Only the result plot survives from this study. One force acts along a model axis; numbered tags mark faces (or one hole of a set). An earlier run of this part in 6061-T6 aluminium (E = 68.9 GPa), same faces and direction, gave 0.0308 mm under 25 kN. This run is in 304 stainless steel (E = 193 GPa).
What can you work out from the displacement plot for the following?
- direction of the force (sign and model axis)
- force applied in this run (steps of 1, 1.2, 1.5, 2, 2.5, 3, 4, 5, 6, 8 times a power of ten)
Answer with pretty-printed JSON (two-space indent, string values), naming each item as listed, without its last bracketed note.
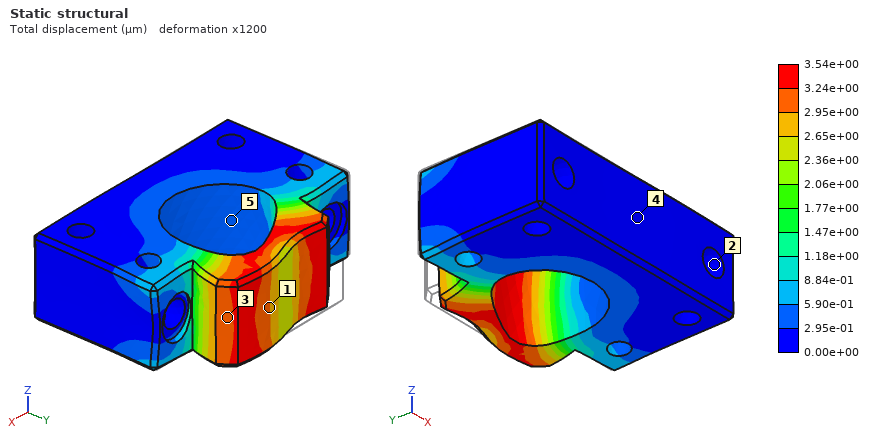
{
  "direction of the force": "+X",
  "force applied in this run": "8 kN"
}
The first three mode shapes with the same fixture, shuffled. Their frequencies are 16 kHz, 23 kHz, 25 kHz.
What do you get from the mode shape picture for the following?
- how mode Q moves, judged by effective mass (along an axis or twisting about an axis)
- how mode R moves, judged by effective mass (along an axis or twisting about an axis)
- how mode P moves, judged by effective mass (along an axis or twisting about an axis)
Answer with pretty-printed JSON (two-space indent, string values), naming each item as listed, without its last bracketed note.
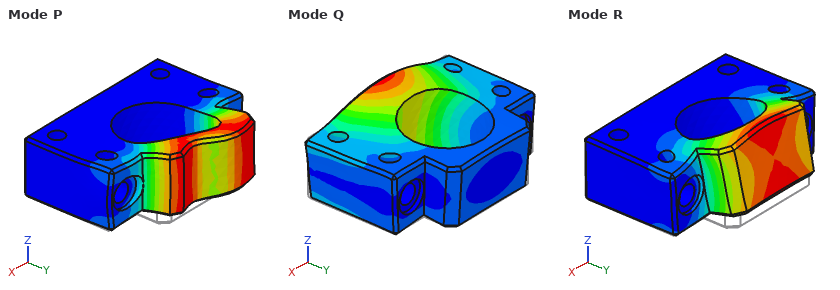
{
  "how mode Q moves, judged by effective mass": "along Z",
  "how mode R moves, judged by effective mass": "along Z",
  "how mode P moves, judged by effective mass": "along X"
}
